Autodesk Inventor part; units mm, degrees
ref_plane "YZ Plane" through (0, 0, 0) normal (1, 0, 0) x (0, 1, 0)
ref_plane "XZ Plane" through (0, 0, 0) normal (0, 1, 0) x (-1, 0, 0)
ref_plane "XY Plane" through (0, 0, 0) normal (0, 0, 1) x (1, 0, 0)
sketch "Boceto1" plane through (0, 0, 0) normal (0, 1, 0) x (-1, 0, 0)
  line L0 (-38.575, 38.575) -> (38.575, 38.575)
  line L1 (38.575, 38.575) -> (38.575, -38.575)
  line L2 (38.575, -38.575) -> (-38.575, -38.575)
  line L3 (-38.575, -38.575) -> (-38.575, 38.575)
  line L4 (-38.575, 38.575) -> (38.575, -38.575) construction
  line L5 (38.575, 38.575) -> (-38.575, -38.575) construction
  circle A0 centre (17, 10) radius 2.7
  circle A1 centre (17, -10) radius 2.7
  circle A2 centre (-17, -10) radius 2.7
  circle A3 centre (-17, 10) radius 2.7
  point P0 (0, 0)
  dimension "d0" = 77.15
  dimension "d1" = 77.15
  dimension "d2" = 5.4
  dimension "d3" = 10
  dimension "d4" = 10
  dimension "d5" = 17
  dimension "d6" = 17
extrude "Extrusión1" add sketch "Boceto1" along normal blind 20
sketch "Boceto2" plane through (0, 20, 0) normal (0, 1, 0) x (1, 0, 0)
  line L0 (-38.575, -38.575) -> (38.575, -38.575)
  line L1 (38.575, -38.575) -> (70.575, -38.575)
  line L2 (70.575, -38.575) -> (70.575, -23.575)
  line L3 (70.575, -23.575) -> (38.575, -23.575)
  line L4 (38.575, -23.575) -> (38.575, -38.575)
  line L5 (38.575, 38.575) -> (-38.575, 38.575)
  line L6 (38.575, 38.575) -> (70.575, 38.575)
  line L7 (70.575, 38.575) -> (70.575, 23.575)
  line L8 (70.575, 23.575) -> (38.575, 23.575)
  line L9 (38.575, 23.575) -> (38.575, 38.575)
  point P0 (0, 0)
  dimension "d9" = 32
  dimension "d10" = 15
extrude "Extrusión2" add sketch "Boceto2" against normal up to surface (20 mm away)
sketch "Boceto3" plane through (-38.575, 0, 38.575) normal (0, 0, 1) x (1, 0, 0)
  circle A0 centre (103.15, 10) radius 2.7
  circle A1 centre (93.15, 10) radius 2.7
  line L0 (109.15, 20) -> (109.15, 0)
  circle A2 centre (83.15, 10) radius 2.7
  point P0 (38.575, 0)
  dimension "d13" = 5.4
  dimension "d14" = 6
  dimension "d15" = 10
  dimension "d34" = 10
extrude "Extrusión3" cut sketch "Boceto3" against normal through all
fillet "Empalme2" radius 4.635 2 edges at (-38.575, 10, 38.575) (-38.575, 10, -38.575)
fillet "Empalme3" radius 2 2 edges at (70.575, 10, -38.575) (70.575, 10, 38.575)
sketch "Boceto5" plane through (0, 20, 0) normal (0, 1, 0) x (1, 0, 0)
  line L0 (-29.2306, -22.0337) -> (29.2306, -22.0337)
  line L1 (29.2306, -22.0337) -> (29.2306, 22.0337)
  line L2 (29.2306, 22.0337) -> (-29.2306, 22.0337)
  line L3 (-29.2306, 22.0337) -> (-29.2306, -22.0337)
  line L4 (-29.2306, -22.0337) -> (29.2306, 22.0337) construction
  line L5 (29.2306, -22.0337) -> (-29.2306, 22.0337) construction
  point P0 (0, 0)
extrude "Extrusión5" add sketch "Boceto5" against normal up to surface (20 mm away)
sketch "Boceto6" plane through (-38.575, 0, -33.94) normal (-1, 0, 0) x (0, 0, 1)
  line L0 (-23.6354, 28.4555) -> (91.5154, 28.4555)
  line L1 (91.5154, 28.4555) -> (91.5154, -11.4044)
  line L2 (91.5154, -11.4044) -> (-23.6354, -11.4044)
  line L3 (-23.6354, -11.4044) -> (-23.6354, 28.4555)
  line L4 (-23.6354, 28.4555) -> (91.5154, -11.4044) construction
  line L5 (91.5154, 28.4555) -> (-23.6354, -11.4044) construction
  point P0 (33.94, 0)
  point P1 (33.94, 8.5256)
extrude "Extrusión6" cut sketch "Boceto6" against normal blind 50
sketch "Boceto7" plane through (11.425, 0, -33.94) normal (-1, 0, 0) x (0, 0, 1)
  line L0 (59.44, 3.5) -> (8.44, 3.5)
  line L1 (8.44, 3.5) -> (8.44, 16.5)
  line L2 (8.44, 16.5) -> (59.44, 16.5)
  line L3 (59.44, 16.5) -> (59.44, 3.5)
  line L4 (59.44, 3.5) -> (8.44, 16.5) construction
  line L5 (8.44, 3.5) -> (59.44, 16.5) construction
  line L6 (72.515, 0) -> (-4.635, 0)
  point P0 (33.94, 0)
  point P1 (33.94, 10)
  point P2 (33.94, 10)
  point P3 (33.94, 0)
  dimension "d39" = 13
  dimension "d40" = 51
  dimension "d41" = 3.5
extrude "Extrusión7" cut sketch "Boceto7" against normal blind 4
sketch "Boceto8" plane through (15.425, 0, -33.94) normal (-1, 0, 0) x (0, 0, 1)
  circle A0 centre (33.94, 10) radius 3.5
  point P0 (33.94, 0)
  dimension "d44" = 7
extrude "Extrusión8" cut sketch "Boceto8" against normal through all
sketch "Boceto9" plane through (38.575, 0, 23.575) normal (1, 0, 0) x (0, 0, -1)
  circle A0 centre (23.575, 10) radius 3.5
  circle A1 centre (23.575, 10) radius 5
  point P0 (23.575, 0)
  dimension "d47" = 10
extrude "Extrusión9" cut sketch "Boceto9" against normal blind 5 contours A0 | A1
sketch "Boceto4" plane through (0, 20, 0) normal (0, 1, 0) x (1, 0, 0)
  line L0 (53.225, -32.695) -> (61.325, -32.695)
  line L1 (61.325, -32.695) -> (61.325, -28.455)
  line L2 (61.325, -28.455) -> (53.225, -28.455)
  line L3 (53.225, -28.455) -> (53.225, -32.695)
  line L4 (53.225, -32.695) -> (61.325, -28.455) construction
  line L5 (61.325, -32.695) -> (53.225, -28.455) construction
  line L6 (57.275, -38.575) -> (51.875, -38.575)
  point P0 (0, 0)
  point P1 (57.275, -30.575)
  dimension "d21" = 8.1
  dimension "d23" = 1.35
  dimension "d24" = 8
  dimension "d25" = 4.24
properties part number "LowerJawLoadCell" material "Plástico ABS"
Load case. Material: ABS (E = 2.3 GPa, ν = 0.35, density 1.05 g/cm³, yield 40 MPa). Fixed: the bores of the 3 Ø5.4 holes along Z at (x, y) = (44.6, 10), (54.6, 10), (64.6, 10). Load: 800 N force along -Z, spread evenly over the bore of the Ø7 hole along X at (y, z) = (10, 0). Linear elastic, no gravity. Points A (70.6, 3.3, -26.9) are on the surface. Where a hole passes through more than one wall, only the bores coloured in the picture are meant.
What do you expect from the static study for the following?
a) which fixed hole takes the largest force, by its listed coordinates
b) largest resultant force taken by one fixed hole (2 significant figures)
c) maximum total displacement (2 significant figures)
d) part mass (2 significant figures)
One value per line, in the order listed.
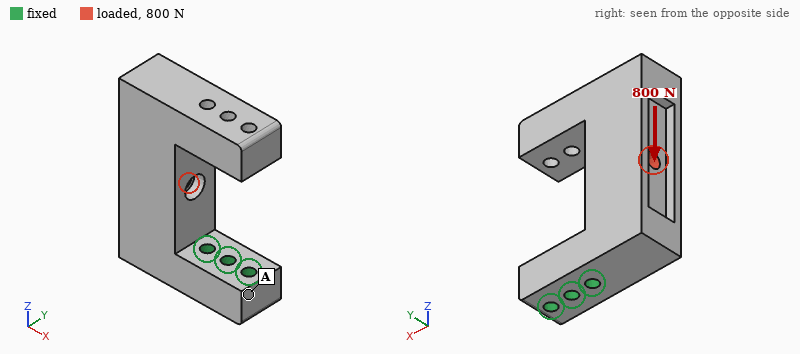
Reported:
(44.6, 10)
960 N
1.0 mm
58 g
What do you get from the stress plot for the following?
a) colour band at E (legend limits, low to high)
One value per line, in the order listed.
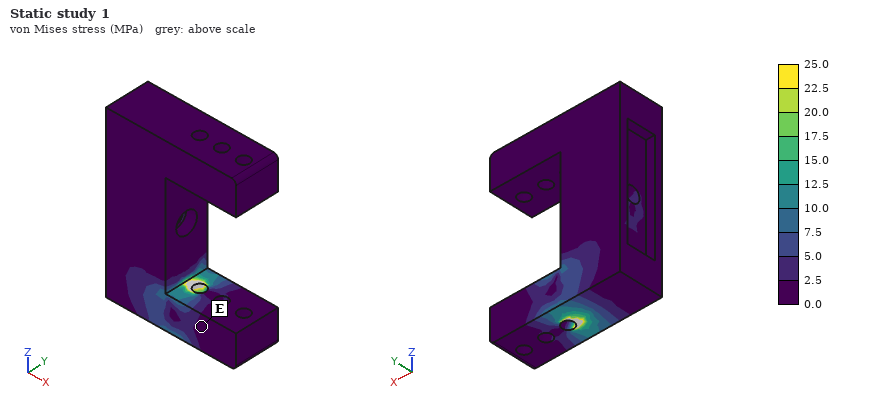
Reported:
0.0 to 2.5 MPa
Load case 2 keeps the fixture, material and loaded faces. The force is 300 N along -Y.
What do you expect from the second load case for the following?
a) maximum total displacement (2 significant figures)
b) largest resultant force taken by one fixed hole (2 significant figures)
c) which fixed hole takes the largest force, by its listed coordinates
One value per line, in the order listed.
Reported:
0.98 mm
530 N
(44.6, 10)
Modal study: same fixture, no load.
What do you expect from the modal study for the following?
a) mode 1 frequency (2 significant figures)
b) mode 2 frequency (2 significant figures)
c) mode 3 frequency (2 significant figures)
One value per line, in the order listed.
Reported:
410 Hz
420 Hz
940 Hz
